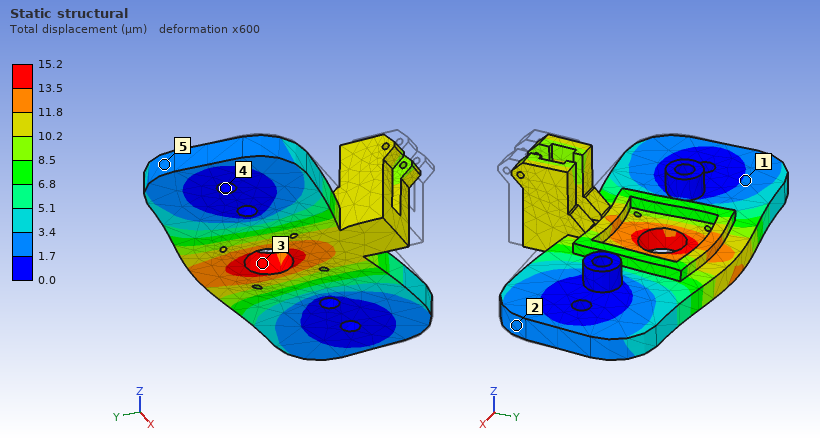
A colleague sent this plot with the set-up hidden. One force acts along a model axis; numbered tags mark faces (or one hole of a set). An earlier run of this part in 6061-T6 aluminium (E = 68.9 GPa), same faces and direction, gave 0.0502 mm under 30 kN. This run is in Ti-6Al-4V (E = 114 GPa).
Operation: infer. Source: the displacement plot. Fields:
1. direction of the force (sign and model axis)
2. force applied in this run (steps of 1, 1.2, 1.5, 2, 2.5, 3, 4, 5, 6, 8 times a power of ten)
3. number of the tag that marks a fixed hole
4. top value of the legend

+Y
15 kN
4
15.2 µm
